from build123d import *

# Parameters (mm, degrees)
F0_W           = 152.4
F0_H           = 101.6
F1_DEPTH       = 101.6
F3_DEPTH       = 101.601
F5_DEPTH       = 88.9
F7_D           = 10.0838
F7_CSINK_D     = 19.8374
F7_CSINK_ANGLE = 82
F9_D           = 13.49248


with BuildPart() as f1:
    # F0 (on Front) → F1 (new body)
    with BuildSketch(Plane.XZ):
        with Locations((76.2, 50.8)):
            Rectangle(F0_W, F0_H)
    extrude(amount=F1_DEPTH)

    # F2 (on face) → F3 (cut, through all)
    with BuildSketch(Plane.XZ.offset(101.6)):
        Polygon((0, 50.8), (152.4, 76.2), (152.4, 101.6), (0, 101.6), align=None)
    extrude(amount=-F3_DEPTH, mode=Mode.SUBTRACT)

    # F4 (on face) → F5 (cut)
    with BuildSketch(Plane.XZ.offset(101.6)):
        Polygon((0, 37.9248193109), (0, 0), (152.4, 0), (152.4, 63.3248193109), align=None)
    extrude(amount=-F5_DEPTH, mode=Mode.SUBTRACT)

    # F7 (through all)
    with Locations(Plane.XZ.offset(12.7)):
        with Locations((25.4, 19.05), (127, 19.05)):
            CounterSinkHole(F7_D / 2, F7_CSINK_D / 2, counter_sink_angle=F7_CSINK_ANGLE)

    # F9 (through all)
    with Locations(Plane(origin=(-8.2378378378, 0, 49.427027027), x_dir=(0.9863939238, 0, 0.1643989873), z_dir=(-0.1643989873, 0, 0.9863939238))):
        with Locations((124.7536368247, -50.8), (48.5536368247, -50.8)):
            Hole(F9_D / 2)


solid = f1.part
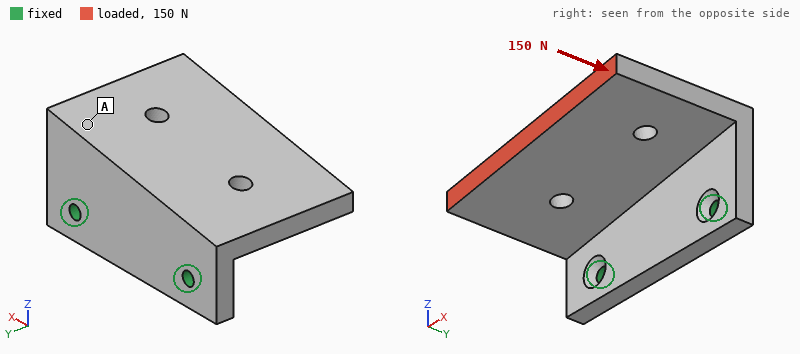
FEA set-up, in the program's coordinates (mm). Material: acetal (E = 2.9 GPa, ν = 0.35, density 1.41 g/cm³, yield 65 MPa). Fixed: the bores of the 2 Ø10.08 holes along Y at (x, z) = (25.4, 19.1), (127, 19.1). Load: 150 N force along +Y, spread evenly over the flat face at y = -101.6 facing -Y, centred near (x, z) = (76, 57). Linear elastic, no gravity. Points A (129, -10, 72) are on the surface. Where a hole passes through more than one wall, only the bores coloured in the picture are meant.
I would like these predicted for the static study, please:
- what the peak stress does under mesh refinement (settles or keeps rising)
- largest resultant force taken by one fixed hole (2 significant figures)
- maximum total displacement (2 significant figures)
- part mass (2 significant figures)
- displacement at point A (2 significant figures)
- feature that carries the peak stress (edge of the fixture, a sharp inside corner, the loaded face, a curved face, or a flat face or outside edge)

keeps rising
75 N
0.37 mm
410 g
0.16 mm
edge of the fixture
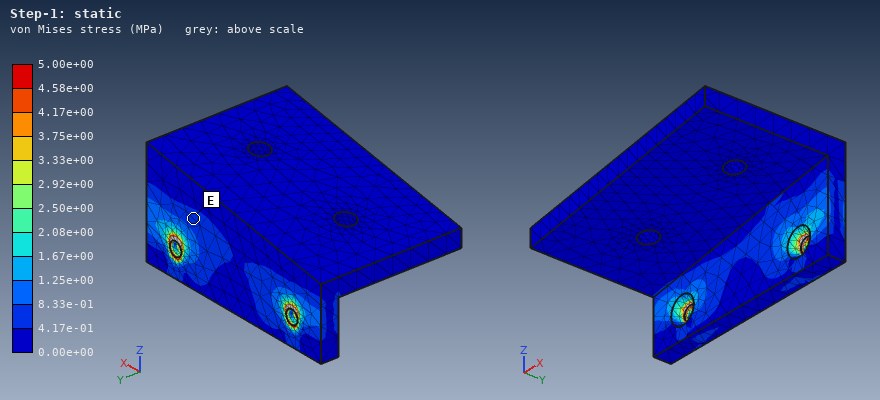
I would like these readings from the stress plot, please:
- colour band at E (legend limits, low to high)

4.17e-01 to 8.33e-01 MPa
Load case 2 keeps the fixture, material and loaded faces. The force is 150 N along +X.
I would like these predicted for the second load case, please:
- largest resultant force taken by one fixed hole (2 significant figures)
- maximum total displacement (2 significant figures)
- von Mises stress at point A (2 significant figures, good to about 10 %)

170 N
0.27 mm
0.80 MPa
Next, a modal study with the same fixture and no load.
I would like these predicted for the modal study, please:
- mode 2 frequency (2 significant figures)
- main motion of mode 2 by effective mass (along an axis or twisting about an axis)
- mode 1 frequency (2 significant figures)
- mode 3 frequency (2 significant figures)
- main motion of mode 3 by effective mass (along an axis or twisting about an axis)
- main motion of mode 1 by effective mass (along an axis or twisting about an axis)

360 Hz
along X
160 Hz
520 Hz
along Y
along Z
